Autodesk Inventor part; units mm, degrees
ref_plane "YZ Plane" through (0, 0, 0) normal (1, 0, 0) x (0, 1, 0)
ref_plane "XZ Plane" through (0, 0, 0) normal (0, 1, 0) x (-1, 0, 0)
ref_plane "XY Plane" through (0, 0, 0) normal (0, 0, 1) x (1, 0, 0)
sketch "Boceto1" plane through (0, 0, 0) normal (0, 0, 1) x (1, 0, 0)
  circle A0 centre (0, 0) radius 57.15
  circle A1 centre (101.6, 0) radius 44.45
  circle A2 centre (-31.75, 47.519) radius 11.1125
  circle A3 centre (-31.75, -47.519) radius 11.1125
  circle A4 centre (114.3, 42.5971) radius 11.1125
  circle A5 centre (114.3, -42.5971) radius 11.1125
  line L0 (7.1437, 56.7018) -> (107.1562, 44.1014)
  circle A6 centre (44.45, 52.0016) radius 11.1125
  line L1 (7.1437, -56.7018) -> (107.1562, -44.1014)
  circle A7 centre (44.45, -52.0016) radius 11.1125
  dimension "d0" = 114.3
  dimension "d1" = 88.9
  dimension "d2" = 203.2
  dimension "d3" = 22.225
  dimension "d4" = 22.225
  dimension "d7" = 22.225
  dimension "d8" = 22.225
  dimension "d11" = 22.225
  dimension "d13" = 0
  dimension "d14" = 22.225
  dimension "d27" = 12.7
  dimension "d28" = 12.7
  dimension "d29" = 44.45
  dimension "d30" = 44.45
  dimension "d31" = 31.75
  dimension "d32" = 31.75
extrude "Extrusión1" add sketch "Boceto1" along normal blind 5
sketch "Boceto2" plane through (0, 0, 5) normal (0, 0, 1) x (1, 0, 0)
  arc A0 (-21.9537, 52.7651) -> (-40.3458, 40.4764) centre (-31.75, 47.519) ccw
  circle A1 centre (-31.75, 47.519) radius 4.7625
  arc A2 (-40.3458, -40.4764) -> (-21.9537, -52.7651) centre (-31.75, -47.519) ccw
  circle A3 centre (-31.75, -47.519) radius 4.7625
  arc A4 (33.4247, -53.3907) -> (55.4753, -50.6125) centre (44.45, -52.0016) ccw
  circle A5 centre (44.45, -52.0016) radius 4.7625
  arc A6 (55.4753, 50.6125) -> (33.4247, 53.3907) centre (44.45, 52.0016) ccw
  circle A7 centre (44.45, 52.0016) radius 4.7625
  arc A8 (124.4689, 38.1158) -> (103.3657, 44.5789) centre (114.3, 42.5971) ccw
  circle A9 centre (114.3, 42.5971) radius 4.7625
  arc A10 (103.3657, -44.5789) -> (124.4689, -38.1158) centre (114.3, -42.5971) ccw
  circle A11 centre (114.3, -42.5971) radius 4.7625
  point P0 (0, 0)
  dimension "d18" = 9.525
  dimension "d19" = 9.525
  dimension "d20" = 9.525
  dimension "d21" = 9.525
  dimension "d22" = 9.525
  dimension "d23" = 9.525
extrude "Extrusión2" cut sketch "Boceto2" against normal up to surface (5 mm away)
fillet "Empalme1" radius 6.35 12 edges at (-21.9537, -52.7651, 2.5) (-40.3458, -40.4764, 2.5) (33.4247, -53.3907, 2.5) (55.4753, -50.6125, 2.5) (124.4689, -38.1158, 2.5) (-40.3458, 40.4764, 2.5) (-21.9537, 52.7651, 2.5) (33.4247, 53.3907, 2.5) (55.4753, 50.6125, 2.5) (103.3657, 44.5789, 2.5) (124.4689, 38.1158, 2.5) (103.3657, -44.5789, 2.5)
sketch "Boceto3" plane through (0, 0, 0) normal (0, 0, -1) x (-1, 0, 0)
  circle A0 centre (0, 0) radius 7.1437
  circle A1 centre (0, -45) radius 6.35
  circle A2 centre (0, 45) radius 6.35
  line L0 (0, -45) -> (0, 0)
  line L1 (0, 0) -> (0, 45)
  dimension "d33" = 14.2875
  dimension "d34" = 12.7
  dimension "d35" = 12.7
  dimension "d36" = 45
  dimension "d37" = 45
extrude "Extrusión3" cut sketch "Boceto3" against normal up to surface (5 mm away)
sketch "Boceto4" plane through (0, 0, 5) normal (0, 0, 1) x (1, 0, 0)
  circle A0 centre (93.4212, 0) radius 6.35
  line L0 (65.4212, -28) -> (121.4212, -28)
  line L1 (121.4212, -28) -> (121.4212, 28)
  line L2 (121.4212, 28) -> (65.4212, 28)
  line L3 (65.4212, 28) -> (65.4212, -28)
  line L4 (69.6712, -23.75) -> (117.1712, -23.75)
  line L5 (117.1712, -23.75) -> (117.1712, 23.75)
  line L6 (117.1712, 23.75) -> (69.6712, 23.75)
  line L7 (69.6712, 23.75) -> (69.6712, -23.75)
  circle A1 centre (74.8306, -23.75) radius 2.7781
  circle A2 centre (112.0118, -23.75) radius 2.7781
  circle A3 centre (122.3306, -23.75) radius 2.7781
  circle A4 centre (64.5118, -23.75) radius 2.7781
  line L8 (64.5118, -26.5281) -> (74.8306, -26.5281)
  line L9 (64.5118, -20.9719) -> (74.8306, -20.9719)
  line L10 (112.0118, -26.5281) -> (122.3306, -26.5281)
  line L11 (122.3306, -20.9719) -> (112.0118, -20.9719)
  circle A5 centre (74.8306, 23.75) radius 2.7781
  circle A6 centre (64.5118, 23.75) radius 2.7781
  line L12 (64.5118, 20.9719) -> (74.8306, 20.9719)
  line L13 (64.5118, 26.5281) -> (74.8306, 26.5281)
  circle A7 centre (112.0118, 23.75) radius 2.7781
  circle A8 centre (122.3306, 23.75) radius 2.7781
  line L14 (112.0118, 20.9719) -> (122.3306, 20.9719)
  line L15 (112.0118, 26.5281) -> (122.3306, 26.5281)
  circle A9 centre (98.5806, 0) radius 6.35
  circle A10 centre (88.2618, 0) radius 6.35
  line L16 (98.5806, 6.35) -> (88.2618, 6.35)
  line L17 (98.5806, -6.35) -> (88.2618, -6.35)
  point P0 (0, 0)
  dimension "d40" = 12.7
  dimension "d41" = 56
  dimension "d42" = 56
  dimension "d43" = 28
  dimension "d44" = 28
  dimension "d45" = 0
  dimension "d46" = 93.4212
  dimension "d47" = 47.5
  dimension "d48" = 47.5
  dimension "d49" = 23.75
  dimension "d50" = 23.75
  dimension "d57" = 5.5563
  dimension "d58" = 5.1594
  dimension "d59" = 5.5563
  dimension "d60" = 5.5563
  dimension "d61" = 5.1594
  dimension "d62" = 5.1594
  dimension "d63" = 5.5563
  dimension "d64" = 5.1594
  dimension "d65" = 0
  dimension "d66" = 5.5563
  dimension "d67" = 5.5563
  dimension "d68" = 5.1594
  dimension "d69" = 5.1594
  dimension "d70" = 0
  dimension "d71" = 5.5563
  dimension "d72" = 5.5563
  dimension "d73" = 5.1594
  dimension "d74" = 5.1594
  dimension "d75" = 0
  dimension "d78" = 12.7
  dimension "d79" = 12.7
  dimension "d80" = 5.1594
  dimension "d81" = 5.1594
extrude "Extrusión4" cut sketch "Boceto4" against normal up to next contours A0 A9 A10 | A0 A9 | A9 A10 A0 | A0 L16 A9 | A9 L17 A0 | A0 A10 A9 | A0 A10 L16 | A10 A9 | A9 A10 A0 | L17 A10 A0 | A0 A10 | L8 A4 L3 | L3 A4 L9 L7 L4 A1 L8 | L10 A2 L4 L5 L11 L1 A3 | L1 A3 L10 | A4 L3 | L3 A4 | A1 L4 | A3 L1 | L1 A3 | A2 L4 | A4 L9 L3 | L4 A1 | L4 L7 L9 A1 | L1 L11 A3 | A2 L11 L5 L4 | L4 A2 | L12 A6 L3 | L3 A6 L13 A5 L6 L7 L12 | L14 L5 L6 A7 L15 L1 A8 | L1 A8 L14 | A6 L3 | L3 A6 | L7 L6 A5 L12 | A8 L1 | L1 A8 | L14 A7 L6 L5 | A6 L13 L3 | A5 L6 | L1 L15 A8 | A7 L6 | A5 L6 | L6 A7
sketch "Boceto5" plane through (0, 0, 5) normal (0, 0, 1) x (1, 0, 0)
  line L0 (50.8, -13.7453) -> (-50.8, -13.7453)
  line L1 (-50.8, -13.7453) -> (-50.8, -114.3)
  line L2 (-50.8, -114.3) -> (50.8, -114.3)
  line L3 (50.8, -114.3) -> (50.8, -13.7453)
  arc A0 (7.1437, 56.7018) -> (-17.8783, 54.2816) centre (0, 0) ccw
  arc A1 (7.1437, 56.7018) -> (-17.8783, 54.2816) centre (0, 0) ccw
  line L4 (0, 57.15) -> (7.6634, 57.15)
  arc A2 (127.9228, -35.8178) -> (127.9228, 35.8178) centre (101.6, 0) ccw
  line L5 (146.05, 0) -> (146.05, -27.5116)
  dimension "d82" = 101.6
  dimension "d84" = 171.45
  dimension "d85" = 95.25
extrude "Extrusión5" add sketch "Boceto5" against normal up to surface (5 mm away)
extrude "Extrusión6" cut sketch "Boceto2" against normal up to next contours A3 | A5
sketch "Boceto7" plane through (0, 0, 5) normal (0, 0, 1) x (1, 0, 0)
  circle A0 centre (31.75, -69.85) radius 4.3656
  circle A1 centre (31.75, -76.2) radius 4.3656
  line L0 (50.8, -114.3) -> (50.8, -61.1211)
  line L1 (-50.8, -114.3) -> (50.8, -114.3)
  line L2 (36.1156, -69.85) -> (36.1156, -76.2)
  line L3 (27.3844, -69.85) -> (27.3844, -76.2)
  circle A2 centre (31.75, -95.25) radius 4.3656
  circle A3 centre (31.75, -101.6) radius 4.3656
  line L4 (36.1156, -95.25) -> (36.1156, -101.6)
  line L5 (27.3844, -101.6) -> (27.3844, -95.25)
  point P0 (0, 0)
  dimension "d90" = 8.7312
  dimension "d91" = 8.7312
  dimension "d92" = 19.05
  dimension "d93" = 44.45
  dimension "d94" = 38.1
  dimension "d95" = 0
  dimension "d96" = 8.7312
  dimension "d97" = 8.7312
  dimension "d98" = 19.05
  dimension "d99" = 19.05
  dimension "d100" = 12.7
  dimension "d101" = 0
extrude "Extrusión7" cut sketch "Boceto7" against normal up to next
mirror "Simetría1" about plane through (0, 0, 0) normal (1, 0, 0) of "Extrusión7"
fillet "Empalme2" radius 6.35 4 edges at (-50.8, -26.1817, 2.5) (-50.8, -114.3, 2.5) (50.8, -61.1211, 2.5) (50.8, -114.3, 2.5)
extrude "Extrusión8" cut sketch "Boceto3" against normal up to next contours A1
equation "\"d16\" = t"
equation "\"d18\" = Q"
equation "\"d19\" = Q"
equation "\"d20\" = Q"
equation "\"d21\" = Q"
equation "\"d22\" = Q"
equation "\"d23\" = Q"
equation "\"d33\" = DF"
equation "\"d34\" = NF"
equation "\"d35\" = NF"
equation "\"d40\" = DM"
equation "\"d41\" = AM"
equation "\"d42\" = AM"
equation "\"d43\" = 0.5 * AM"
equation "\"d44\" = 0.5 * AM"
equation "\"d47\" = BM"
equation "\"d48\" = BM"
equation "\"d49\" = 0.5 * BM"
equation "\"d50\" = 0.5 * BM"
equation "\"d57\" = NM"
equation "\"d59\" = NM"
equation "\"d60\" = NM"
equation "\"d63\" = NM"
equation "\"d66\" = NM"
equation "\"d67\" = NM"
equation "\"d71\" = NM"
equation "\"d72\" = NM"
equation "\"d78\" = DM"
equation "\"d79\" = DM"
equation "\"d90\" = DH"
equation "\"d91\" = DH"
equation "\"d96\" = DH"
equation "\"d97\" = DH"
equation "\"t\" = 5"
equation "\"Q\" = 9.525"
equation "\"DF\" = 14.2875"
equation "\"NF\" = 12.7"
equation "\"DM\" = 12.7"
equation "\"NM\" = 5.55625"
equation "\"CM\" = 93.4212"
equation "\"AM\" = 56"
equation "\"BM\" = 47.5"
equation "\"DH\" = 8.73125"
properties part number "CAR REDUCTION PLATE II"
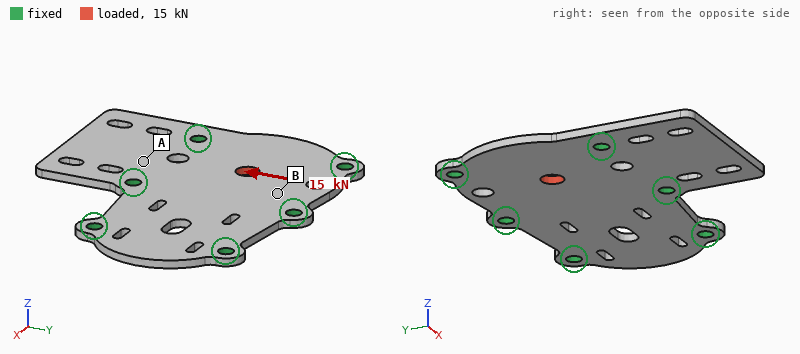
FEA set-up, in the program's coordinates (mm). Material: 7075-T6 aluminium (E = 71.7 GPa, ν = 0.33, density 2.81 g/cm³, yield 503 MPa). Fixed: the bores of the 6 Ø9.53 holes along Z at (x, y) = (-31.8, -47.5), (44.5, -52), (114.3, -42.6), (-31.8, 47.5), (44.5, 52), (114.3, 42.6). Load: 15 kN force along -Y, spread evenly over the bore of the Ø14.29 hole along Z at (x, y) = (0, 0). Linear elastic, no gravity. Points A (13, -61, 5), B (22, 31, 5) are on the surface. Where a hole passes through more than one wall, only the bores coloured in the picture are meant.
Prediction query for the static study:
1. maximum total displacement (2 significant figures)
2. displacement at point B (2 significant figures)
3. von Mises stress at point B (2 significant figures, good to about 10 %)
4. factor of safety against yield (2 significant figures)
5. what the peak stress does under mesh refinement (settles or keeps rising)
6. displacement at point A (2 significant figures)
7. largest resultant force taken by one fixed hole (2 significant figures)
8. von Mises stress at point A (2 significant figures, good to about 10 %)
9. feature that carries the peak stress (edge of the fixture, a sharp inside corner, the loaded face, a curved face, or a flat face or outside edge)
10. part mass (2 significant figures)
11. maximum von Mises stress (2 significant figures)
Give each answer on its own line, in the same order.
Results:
31 µm
13 µm
24 MPa
4.3
settles
8.2 µm
4.8 kN
9.8 MPa
the loaded face
340 g
120 MPa
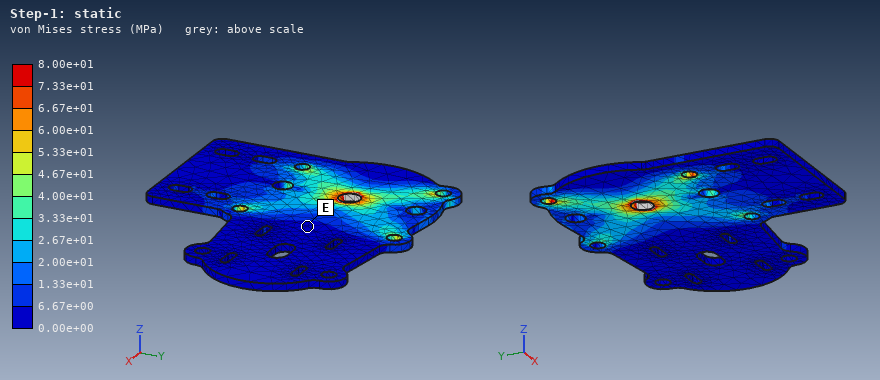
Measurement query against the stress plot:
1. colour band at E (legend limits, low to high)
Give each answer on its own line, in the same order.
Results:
0.00e+00 to 6.67e+00 MPa
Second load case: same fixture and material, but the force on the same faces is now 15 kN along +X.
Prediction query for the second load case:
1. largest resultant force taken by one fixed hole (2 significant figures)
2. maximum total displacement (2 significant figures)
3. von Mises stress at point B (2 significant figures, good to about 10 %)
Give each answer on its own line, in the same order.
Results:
3.8 kN
37 µm
23 MPa
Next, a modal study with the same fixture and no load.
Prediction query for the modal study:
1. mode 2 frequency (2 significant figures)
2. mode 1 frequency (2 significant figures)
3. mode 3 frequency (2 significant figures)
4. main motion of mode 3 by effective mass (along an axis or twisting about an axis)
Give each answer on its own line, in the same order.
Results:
1800 Hz
940 Hz
2400 Hz
along Z
